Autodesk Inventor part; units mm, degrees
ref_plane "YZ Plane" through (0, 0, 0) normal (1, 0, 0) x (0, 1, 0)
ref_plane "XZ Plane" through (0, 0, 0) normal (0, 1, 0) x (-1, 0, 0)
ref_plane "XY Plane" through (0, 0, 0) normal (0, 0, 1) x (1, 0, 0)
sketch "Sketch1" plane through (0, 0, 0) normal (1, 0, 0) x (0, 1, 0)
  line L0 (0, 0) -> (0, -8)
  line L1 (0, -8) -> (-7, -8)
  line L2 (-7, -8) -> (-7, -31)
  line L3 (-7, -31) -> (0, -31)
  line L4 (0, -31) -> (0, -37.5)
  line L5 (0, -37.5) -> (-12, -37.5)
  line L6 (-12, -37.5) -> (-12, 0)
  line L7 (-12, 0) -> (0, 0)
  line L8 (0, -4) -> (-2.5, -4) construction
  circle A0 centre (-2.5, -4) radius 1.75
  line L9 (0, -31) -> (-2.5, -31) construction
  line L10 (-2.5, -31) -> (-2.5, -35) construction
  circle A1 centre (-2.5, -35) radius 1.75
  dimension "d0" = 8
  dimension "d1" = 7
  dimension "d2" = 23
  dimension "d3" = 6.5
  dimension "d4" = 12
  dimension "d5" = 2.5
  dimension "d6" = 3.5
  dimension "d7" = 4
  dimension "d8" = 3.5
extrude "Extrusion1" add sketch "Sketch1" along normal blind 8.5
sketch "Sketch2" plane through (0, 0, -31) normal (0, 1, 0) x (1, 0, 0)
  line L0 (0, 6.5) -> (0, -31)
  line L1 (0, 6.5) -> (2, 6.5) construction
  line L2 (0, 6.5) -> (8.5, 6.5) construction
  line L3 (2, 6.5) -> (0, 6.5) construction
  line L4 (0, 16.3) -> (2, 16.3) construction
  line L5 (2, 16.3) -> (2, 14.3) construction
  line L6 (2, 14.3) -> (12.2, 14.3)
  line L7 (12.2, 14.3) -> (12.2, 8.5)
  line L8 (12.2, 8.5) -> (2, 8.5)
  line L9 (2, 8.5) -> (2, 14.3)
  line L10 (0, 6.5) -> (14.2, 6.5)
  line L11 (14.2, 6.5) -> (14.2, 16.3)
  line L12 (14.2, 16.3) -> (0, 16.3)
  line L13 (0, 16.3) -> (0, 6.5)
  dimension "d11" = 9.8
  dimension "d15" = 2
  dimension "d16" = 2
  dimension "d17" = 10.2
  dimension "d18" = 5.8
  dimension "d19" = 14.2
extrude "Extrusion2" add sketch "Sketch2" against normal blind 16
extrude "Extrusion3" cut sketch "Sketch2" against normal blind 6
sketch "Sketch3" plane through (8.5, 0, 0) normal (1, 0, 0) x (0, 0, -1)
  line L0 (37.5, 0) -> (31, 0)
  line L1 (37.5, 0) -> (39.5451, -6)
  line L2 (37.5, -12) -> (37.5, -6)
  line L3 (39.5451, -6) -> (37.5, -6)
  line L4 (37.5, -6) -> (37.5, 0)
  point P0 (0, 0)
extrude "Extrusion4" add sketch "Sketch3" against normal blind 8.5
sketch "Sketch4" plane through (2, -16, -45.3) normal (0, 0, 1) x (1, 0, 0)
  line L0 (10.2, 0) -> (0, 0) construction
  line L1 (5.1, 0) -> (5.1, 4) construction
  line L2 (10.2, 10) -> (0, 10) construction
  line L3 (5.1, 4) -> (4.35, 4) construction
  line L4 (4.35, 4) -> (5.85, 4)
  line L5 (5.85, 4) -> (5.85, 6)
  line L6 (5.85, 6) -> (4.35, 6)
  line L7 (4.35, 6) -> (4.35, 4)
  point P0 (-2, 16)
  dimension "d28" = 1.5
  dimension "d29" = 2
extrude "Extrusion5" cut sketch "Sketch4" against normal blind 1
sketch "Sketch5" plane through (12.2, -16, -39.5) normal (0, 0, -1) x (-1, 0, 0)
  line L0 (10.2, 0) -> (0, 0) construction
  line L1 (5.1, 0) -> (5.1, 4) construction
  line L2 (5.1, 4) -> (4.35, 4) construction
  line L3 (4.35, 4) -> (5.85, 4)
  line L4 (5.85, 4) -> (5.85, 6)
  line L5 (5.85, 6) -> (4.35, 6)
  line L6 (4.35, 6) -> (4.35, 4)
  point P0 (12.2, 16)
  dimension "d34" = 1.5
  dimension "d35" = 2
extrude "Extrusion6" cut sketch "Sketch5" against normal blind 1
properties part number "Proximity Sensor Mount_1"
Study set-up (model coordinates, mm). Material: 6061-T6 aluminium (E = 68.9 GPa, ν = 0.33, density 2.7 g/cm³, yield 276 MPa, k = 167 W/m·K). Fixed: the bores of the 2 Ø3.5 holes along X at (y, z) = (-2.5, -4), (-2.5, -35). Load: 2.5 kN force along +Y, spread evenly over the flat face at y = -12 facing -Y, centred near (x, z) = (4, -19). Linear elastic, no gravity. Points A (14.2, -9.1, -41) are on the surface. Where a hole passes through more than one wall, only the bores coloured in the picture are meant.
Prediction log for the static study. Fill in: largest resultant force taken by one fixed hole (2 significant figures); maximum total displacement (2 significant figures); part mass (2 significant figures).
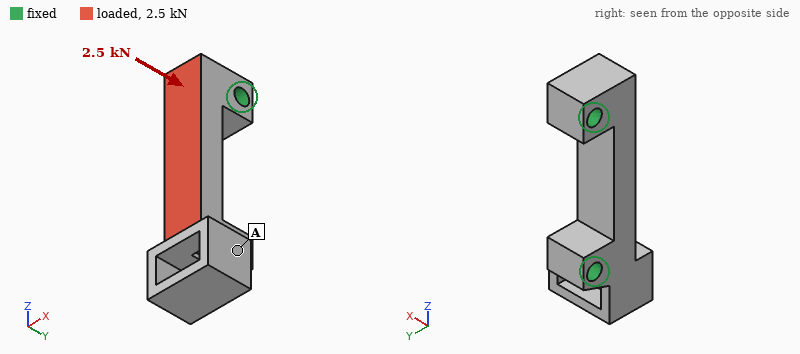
1.4 kN
26 µm
8.5 g
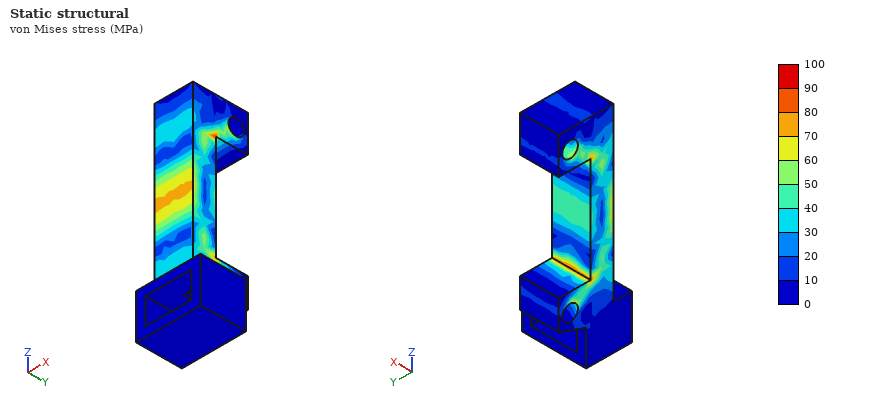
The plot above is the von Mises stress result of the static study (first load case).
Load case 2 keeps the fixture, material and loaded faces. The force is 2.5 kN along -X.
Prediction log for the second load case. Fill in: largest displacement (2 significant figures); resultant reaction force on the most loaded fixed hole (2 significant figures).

43 µm
1.3 kN
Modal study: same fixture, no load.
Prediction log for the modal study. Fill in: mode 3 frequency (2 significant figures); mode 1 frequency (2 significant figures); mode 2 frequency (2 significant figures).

22 kHz
11 kHz
13 kHz
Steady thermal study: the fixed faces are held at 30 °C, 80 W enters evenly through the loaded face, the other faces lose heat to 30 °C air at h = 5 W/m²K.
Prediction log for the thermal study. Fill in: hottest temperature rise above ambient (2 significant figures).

48 K
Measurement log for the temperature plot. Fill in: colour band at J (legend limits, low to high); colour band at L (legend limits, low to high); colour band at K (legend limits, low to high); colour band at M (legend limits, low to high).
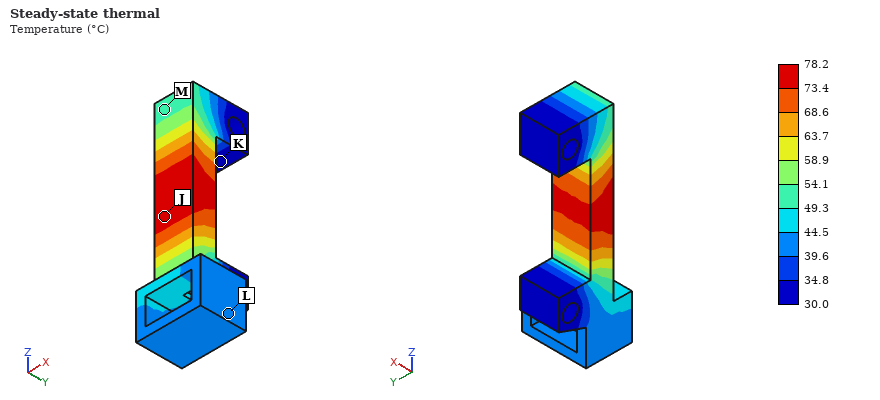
73.4 to 78.2 °C
39.6 to 44.5 °C
30.0 to 34.8 °C
49.3 to 54.1 °C
